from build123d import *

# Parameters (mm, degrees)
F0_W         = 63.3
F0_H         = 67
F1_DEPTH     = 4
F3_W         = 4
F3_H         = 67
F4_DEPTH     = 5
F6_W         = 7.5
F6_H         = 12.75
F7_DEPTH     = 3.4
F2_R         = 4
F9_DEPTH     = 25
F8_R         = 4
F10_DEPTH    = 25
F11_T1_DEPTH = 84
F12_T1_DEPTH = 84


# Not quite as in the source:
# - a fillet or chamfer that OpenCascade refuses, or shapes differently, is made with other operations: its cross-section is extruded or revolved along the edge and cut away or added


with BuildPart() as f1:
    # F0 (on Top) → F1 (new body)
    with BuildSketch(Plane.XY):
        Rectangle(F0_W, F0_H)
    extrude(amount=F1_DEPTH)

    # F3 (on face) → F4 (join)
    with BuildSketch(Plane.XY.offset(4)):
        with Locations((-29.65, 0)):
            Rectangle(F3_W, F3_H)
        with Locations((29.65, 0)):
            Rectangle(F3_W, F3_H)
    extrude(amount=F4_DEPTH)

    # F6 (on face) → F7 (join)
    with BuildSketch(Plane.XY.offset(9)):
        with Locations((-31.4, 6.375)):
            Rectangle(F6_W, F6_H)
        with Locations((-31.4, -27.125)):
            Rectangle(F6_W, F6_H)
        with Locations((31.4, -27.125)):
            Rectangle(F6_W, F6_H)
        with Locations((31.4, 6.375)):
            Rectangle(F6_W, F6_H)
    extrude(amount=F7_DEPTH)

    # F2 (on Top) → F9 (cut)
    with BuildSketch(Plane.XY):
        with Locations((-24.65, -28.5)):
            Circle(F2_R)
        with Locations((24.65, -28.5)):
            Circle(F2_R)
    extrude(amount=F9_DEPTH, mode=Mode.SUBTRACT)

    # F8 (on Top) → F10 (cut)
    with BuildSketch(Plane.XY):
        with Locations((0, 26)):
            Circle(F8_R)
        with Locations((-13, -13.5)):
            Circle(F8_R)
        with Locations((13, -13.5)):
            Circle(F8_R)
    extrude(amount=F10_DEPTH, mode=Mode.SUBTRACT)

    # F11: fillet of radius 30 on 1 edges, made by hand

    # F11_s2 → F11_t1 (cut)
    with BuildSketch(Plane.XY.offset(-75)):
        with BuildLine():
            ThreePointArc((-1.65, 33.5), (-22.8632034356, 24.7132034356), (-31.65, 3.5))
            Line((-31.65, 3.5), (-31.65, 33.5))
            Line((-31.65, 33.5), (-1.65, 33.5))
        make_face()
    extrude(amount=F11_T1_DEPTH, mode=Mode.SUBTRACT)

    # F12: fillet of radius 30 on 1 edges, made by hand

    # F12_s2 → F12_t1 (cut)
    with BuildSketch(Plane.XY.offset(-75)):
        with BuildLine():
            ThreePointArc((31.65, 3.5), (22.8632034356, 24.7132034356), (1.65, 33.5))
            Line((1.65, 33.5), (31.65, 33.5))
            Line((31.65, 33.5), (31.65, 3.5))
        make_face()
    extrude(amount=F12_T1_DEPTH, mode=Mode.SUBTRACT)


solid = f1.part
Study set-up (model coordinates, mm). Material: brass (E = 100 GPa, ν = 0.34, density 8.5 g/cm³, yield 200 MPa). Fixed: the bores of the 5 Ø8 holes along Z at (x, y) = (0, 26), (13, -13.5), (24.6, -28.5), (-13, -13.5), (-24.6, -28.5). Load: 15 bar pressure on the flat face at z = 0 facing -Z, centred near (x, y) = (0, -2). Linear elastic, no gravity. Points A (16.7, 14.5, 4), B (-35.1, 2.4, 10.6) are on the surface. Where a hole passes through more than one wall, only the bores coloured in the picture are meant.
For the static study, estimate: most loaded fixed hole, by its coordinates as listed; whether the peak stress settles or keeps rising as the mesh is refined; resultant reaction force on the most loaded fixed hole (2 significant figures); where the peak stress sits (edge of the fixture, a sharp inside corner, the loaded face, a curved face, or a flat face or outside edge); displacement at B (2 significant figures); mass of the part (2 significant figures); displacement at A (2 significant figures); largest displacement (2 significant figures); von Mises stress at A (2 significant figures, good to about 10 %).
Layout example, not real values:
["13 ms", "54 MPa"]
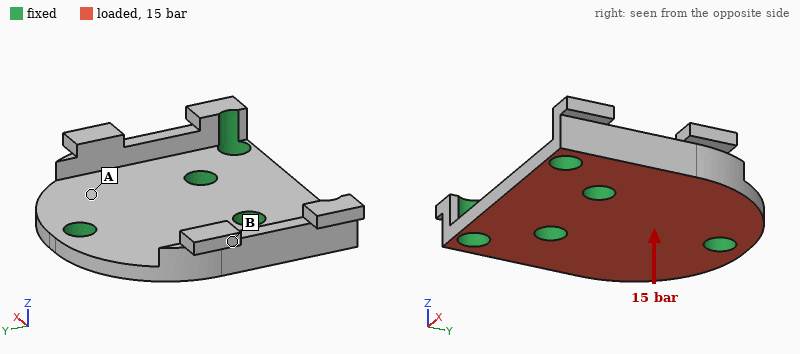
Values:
["(0, 26)", "keeps rising", "1.6 kN", "edge of the fixture", "50 µm", "150 g", "34 µm", "71 µm", "32 MPa"]
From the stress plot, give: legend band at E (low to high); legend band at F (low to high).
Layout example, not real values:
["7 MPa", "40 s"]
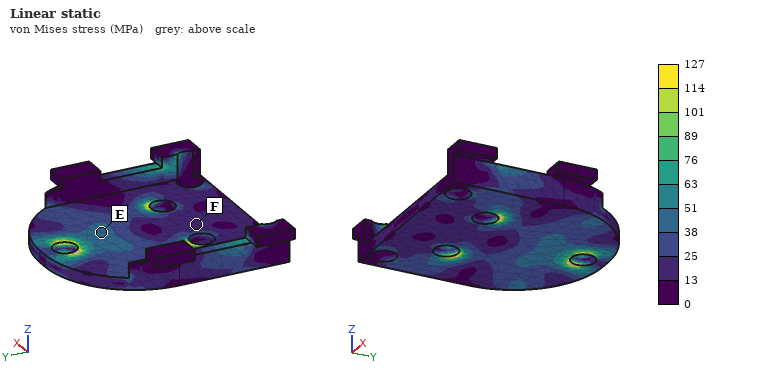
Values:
["38 to 51 MPa", "13 to 25 MPa"]
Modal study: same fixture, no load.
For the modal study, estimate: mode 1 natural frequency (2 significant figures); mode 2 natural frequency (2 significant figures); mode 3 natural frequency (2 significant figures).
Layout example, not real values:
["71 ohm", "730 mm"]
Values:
["4200 Hz", "4300 Hz", "8900 Hz"]
